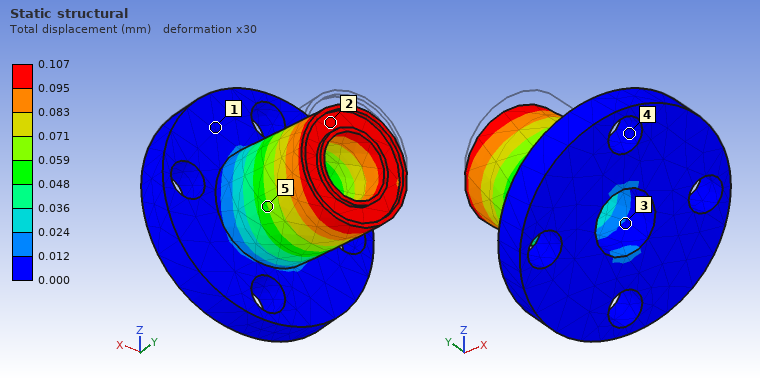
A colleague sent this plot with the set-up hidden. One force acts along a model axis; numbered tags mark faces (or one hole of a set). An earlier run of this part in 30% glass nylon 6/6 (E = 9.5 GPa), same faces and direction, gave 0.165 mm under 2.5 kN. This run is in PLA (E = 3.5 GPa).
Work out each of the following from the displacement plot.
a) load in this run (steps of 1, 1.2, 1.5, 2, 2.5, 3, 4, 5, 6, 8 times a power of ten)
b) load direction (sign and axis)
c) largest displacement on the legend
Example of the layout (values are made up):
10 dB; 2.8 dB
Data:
600 N; -Z; 0.107 mm
